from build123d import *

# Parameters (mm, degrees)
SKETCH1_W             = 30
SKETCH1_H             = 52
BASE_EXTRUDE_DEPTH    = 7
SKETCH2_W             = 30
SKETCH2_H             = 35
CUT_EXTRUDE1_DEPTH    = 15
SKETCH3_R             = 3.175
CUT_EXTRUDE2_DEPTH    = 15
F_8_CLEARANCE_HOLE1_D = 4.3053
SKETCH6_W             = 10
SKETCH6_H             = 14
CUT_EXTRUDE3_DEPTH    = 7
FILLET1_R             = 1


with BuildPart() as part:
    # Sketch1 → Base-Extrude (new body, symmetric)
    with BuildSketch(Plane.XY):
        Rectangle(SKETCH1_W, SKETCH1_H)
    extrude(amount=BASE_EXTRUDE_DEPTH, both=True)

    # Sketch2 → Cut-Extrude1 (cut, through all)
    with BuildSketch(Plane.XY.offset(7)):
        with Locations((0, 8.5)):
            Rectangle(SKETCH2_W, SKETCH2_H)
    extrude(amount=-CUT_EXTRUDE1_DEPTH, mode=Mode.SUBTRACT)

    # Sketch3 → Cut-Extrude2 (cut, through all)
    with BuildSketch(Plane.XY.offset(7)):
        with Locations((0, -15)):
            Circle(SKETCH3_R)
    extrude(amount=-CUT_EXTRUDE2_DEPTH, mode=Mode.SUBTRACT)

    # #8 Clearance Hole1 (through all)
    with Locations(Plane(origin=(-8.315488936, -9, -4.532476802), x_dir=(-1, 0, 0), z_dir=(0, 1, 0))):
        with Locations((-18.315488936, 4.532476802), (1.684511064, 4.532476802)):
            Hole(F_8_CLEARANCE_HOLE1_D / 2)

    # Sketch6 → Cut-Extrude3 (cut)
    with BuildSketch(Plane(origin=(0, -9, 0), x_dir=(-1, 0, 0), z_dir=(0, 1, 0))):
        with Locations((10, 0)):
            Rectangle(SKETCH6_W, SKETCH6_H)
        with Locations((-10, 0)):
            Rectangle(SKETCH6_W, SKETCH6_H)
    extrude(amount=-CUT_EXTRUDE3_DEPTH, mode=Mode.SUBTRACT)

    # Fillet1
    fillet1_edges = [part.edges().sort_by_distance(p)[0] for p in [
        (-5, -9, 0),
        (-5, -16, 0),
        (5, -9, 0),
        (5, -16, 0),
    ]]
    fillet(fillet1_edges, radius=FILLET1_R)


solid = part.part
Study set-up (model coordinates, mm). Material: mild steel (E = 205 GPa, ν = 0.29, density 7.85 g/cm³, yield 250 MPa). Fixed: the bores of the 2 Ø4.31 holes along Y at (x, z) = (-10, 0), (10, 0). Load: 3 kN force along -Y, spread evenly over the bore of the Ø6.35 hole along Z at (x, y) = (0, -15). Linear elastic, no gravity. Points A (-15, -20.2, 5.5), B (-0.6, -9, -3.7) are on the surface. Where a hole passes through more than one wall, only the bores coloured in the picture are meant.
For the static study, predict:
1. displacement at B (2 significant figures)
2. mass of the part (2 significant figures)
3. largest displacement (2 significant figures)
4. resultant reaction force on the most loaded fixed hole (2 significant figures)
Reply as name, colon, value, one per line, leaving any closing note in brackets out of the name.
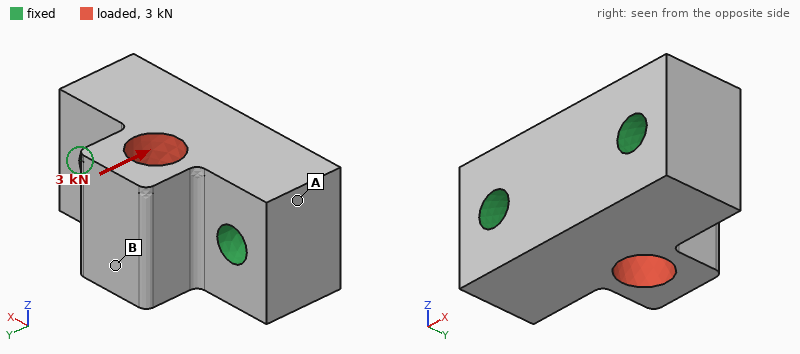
displacement at B: 2.0 µm
mass of the part: 35 g
largest displacement: 2.1 µm
resultant reaction force on the most loaded fixed hole: 1.5 kN
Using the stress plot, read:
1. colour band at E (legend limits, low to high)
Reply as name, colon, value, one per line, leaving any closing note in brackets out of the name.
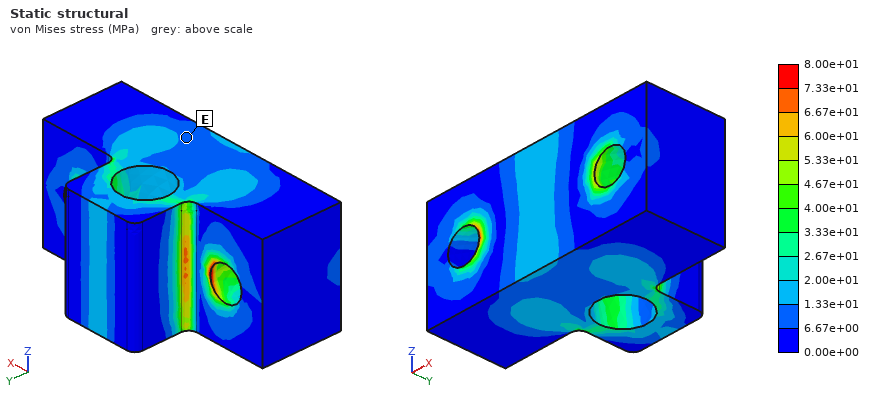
colour band at E: 6.67e+00 to 1.33e+01 MPa
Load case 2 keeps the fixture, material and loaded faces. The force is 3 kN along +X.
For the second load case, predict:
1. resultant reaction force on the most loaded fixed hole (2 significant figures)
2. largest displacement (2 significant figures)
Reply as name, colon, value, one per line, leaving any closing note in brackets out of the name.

resultant reaction force on the most loaded fixed hole: 1.7 kN
largest displacement: 4.5 µm
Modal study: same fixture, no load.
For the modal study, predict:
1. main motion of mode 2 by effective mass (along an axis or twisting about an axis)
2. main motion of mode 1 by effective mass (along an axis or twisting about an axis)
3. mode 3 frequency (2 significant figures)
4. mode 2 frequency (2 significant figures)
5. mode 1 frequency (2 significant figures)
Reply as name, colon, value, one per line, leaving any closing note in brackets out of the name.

main motion of mode 2 by effective mass: along X
main motion of mode 1 by effective mass: along Z
mode 3 frequency: 56 kHz
mode 2 frequency: 43 kHz
mode 1 frequency: 36 kHz
